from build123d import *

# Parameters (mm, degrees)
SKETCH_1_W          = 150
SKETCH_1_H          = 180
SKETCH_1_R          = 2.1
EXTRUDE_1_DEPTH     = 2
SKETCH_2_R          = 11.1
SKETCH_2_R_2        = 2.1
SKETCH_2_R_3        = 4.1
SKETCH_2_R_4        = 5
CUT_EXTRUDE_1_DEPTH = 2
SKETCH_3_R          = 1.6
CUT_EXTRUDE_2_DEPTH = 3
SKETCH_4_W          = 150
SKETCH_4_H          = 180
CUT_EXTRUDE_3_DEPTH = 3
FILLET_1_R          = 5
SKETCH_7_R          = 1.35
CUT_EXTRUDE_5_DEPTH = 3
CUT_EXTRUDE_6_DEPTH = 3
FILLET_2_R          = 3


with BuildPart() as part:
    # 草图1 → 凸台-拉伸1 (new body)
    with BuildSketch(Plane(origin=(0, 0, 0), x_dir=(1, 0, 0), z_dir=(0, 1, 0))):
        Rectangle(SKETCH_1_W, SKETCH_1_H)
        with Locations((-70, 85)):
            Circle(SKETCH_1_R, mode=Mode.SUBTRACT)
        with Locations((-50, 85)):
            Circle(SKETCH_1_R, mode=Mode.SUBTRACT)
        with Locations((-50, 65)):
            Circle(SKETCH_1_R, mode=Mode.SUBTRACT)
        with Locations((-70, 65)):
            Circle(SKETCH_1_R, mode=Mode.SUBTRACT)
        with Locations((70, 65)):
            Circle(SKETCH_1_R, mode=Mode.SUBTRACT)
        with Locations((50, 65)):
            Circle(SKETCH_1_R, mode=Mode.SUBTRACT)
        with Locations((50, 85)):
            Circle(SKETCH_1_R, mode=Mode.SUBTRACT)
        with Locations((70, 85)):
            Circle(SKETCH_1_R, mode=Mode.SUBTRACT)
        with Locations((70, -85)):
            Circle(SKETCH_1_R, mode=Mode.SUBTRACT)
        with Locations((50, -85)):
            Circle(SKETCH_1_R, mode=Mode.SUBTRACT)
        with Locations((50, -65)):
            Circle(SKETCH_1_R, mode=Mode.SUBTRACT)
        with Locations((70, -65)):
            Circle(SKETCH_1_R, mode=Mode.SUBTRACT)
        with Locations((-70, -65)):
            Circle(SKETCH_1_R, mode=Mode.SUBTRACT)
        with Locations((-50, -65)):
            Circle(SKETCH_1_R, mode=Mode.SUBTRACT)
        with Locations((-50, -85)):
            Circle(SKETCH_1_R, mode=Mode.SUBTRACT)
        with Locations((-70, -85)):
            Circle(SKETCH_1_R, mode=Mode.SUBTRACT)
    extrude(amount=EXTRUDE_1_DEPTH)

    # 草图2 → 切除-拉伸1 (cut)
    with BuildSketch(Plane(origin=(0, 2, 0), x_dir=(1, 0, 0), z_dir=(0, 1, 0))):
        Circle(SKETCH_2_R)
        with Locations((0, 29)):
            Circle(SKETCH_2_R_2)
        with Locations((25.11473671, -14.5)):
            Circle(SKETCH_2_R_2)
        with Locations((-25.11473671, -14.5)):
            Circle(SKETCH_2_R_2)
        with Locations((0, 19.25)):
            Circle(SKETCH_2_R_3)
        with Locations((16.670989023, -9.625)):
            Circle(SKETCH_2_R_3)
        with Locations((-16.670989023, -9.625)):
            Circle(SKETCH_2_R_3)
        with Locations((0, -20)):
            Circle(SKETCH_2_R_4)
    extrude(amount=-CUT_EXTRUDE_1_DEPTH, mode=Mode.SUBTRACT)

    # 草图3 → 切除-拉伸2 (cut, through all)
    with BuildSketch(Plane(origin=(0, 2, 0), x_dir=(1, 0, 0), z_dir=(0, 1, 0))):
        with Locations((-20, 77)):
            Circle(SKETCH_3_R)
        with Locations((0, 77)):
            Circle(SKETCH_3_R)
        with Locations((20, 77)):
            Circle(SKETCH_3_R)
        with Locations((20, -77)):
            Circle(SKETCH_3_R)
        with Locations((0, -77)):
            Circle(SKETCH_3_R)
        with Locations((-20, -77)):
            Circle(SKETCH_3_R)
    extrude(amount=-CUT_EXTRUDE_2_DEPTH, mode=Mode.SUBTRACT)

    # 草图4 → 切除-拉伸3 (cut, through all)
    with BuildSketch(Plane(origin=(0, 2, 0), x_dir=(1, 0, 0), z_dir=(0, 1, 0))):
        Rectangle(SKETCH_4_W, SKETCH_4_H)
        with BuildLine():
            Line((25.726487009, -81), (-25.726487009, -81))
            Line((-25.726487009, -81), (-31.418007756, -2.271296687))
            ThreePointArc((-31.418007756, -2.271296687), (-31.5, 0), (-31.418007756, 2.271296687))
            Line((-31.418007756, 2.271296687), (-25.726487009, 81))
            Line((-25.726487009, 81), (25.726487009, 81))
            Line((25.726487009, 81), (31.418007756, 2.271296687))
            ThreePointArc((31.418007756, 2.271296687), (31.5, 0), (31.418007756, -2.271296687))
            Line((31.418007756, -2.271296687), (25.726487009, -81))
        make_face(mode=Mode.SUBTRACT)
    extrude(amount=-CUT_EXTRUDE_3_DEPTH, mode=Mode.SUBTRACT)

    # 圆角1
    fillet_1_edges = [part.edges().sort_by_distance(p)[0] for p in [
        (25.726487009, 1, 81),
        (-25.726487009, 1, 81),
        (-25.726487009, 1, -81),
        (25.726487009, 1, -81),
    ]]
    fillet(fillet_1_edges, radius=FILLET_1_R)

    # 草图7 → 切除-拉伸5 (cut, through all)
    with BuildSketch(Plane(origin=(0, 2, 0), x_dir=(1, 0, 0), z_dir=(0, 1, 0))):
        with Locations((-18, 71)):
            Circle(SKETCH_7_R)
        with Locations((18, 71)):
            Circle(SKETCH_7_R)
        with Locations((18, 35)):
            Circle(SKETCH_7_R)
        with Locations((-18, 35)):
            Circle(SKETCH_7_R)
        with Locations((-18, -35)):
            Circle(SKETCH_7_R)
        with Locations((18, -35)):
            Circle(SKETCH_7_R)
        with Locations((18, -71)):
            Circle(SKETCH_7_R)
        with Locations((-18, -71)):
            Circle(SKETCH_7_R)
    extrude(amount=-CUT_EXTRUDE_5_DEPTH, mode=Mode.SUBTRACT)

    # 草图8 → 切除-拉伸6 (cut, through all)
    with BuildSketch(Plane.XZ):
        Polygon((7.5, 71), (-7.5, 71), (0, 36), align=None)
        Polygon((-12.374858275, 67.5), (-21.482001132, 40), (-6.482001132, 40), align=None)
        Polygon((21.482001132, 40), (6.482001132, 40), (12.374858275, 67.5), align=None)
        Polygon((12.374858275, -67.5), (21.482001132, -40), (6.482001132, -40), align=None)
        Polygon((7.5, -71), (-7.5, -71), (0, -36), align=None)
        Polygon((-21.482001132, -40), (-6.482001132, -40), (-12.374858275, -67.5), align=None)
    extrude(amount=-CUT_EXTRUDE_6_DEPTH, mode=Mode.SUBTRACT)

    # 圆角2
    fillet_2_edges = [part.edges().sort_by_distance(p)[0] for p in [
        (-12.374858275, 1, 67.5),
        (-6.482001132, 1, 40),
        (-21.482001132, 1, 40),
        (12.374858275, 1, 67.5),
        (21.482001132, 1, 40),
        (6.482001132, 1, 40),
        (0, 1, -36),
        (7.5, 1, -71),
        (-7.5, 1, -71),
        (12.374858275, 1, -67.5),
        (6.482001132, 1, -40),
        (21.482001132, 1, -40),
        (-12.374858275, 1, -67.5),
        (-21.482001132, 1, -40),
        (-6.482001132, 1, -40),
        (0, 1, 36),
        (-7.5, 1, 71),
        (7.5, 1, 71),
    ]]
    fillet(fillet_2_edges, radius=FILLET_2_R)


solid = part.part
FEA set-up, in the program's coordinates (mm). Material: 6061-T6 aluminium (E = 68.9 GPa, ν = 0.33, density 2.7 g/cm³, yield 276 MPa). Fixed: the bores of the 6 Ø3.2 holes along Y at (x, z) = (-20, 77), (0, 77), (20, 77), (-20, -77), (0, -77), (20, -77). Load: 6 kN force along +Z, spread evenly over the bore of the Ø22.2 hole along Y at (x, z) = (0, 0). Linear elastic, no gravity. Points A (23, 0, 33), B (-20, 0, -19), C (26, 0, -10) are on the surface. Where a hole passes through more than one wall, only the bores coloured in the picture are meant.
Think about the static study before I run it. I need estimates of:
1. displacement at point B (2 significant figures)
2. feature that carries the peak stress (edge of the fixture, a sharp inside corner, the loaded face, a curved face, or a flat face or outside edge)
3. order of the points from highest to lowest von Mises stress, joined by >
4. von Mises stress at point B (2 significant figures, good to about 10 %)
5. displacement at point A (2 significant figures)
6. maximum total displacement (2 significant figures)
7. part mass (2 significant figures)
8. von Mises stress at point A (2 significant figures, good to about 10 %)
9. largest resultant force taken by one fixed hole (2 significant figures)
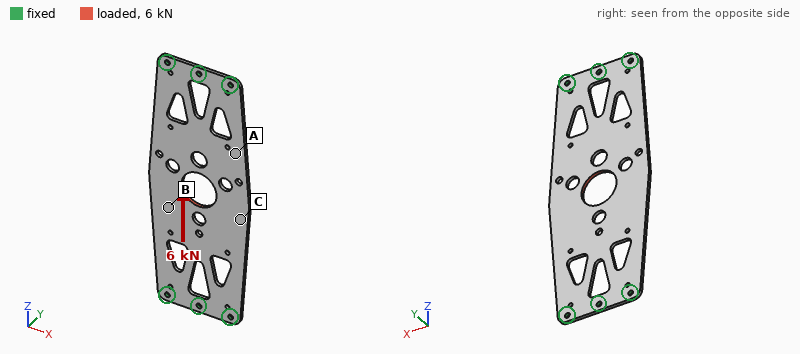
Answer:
40 µm
a curved face
A > B > C
26 MPa
31 µm
60 µm
40 g
34 MPa
1.3 kN
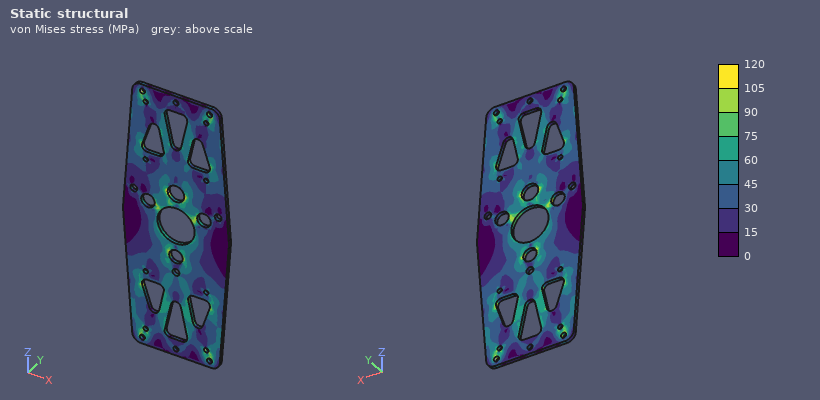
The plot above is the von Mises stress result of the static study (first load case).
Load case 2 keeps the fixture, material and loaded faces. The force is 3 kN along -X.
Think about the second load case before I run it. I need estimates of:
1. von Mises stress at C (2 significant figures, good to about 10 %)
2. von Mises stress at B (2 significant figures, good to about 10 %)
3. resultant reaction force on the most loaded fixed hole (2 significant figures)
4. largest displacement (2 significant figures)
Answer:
45 MPa
28 MPa
1.1 kN
0.15 mm
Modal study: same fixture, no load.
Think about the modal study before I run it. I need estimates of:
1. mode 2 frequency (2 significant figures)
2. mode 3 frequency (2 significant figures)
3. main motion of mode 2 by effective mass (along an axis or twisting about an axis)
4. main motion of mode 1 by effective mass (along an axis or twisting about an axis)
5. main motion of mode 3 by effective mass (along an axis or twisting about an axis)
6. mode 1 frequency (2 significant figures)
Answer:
710 Hz
1200 Hz
twisting about Z
along Y
twisting about X
400 Hz
